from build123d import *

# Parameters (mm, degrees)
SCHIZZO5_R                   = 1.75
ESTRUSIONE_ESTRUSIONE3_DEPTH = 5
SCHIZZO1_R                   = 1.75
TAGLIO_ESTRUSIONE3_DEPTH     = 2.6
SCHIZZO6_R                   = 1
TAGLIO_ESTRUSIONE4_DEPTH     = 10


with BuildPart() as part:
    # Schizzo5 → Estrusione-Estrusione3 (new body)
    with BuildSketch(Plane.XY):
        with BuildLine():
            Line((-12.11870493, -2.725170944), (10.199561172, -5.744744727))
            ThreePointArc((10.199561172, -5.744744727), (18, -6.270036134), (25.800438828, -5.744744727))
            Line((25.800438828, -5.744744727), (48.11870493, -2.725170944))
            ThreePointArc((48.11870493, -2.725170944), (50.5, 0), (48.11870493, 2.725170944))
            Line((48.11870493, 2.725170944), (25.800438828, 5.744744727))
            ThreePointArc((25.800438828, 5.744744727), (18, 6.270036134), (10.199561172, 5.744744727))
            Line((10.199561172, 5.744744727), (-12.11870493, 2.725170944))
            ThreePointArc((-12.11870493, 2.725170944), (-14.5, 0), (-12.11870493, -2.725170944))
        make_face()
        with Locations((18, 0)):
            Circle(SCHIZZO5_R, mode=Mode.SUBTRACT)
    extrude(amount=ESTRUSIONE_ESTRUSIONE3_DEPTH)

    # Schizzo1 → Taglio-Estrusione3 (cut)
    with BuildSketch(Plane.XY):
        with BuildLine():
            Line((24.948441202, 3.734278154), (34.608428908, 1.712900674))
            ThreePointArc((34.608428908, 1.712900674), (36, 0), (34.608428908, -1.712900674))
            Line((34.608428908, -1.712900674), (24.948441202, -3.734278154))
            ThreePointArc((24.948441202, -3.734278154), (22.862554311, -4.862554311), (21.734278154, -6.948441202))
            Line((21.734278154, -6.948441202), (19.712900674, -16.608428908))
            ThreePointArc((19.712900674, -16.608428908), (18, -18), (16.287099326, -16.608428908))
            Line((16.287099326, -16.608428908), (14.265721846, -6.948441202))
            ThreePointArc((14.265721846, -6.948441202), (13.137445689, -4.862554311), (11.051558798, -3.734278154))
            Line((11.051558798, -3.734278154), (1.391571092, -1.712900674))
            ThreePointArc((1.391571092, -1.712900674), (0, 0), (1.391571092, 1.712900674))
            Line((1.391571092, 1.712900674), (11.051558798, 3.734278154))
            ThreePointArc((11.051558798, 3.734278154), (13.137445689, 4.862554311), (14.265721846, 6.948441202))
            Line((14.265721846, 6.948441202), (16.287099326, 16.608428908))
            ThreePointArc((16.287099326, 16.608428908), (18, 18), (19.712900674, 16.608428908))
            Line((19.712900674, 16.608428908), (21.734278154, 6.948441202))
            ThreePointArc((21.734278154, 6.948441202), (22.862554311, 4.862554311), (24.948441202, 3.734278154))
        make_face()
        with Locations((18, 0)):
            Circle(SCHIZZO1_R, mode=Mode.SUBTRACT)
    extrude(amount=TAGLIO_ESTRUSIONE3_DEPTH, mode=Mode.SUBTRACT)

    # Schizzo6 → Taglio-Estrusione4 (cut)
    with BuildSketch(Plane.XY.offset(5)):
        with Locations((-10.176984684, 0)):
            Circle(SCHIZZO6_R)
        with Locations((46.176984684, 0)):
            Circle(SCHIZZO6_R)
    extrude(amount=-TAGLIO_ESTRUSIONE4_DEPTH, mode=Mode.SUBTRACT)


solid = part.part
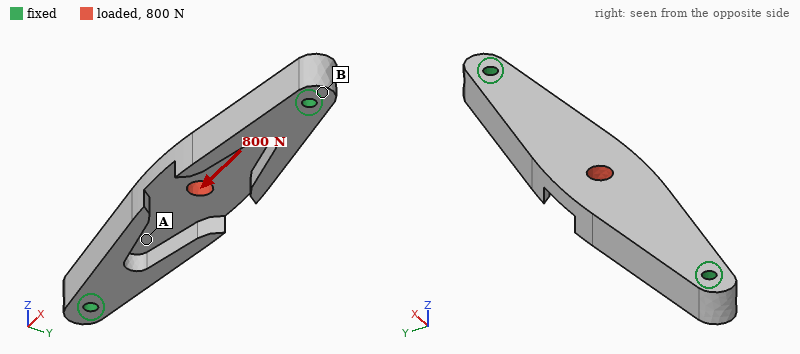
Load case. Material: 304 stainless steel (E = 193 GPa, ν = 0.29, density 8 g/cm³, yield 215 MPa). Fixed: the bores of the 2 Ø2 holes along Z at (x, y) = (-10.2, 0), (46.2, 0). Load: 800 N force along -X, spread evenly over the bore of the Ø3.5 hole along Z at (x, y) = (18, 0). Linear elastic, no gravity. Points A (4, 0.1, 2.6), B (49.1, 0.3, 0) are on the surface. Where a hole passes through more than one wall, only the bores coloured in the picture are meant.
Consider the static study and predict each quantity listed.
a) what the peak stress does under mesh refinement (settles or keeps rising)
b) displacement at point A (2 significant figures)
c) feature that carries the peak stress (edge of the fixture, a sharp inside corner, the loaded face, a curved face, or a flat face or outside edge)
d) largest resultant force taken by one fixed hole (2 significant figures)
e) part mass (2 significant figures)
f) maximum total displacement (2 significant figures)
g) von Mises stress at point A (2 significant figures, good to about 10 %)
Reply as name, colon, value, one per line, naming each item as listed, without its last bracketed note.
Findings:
what the peak stress does under mesh refinement: keeps rising
displacement at point A: 0.86 µm
feature that carries the peak stress: a sharp inside corner
largest resultant force taken by one fixed hole: 400 N
part mass: 18 g
maximum total displacement: 2.2 µm
von Mises stress at point A: 12 MPa
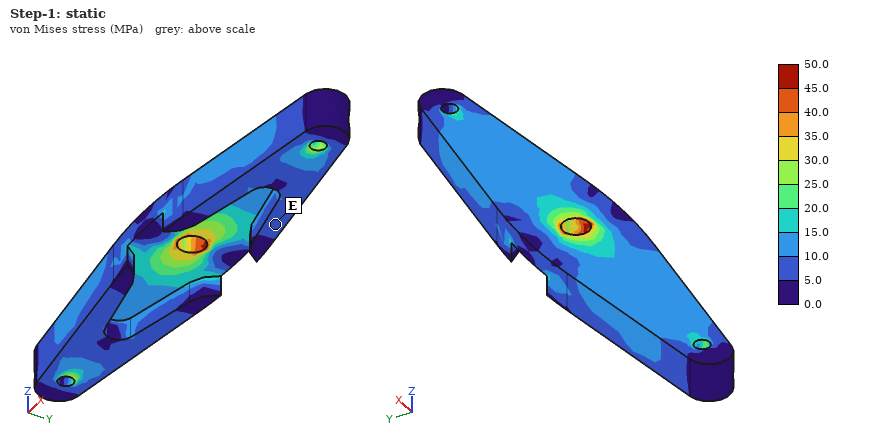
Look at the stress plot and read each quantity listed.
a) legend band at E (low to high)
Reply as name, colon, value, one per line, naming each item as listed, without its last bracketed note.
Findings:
legend band at E: 5.0 to 10.0 MPa
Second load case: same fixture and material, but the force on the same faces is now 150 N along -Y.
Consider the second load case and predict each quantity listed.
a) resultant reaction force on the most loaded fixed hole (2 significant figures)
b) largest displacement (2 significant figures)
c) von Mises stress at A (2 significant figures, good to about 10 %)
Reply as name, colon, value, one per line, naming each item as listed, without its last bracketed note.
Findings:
resultant reaction force on the most loaded fixed hole: 75 N
largest displacement: 5.5 µm
von Mises stress at A: 4.8 MPa
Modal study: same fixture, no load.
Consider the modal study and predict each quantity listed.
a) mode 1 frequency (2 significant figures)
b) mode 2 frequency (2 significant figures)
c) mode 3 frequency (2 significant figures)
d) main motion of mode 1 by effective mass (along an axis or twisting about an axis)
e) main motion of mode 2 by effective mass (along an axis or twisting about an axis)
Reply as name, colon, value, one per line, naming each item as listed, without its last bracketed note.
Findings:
mode 1 frequency: 6500 Hz
mode 2 frequency: 10 kHz
mode 3 frequency: 15 kHz
main motion of mode 1 by effective mass: along Z
main motion of mode 2 by effective mass: along Y
